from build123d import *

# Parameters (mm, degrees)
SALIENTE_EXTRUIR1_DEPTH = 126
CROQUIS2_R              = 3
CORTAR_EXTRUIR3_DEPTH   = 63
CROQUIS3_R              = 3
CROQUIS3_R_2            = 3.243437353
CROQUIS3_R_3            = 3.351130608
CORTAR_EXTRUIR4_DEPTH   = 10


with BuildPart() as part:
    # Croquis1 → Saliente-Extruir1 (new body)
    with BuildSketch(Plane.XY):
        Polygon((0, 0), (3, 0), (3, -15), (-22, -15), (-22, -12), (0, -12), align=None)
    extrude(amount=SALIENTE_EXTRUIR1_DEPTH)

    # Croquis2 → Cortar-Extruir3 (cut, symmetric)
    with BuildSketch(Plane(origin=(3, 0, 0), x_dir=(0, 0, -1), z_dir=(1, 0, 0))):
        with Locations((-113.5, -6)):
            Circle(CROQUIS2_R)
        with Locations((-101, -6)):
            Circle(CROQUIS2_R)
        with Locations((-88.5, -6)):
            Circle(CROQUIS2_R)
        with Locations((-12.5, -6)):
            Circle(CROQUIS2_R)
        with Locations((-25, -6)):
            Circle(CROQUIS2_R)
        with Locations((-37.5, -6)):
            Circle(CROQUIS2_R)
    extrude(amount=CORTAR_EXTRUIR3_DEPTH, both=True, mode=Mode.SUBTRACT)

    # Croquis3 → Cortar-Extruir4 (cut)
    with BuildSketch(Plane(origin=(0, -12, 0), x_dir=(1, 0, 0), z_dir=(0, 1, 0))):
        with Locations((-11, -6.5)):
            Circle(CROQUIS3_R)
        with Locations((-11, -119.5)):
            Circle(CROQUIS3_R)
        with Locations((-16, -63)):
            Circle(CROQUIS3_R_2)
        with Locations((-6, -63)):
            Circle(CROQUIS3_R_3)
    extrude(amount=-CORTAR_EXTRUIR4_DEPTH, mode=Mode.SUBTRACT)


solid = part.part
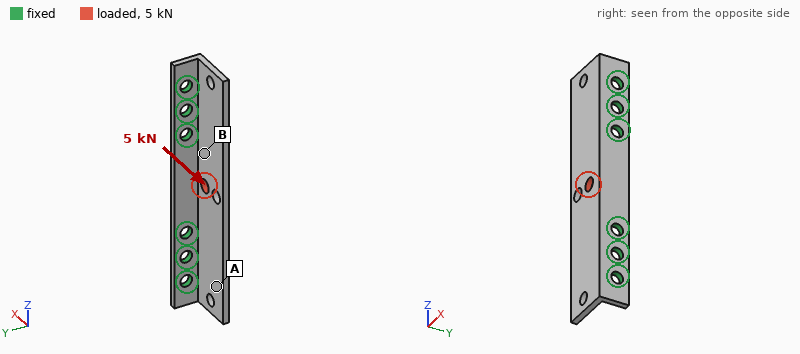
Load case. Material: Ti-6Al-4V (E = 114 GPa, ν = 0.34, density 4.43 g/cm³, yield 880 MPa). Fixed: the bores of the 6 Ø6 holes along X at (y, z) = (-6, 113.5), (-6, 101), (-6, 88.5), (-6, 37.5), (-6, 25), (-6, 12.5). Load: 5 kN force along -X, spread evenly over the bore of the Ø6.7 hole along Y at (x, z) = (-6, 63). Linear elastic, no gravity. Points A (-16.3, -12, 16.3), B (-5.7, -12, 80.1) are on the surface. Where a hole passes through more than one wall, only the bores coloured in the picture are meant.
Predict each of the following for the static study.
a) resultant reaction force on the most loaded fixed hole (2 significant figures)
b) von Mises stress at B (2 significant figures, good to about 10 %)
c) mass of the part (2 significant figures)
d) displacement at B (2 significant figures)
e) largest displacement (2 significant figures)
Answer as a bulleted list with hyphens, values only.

- 2.2 kN
- 70 MPa
- 58 g
- 0.057 mm
- 0.15 mm
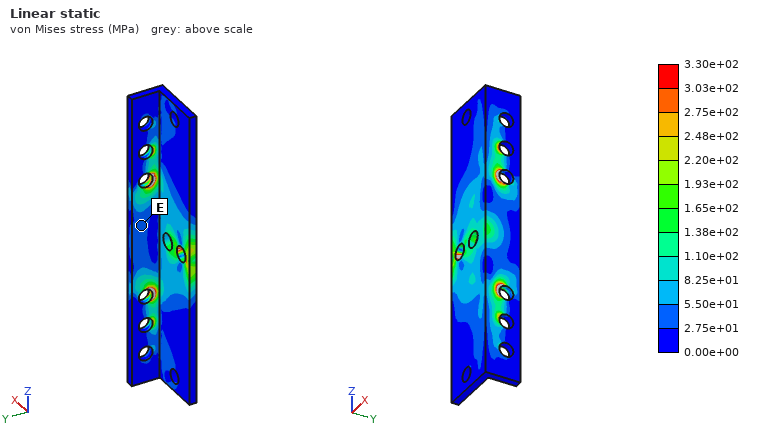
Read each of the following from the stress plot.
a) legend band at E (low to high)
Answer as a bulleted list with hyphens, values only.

- 2.75e+01 to 5.50e+01 MPa
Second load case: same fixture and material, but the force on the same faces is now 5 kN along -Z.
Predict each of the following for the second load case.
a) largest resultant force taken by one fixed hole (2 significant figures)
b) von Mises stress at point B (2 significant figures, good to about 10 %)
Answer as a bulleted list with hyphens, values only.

- 1.7 kN
- 35 MPa
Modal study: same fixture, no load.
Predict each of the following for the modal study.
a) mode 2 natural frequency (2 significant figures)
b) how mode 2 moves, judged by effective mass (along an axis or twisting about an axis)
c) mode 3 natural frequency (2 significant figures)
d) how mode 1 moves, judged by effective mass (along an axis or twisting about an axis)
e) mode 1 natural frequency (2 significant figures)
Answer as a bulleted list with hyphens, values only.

- 3800 Hz
- twisting about X
- 4800 Hz
- along Y
- 3200 Hz
